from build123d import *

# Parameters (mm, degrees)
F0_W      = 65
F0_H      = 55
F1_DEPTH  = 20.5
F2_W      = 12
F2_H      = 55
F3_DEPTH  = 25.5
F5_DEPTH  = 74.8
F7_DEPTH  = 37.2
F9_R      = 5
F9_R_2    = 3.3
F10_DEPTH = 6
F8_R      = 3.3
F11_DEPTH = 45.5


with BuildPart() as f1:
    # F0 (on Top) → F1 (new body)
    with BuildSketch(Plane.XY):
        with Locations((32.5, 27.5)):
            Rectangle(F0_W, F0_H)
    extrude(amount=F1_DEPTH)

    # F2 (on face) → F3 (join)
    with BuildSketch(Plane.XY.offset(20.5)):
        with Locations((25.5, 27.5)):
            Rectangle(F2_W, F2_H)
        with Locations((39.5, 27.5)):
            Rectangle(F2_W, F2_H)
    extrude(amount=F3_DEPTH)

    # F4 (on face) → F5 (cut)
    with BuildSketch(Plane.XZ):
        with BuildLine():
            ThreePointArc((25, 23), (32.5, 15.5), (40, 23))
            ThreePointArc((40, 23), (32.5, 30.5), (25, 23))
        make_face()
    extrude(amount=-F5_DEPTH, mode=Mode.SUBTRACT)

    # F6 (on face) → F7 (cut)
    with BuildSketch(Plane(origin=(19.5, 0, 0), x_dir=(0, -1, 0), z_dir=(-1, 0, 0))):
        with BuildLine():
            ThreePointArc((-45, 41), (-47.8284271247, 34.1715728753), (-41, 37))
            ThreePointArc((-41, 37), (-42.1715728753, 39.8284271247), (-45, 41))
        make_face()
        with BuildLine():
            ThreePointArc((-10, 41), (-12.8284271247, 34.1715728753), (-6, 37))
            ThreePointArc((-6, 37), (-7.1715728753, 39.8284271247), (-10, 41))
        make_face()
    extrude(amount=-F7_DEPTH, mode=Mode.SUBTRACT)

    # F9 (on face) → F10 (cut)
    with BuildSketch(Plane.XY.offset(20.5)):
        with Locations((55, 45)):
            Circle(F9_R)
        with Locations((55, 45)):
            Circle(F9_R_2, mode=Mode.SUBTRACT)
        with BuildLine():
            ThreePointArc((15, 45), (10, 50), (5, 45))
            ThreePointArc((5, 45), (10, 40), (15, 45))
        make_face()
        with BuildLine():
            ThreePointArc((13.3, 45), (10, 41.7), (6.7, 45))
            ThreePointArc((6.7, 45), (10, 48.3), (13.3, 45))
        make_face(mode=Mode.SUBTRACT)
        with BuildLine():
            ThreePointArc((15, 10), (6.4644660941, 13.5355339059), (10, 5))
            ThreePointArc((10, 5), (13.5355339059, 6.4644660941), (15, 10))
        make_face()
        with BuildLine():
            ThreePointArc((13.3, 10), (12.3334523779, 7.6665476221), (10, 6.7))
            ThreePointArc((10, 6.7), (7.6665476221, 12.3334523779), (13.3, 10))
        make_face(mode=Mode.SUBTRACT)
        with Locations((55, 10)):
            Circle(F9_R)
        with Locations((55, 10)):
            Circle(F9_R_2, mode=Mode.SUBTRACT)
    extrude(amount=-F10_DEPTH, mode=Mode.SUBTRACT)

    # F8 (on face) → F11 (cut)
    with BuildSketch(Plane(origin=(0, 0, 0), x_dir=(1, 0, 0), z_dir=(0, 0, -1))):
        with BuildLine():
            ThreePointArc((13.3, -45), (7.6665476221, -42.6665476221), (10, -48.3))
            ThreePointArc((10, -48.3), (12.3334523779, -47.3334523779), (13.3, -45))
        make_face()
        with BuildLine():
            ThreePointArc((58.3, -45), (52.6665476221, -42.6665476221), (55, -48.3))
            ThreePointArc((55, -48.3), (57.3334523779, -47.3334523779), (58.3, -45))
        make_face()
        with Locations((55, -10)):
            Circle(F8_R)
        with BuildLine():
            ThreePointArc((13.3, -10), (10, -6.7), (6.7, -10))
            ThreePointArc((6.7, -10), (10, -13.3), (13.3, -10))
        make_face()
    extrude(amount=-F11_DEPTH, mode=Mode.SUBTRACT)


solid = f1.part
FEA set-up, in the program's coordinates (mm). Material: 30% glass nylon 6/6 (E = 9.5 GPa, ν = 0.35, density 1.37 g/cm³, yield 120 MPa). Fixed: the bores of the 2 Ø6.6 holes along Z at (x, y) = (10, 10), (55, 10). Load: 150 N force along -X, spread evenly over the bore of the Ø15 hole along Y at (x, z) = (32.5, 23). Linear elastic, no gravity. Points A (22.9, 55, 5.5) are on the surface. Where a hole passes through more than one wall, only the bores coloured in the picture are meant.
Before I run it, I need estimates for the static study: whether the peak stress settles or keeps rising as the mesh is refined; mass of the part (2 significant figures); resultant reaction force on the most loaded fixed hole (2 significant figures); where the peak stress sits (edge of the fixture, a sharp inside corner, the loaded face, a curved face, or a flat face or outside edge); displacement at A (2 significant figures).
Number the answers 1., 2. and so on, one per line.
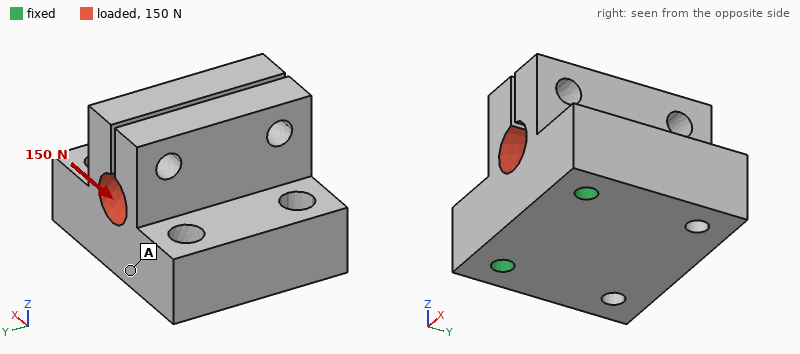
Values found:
1. keeps rising
2. 130 g
3. 100 N
4. edge of the fixture
5. 1.2 µm
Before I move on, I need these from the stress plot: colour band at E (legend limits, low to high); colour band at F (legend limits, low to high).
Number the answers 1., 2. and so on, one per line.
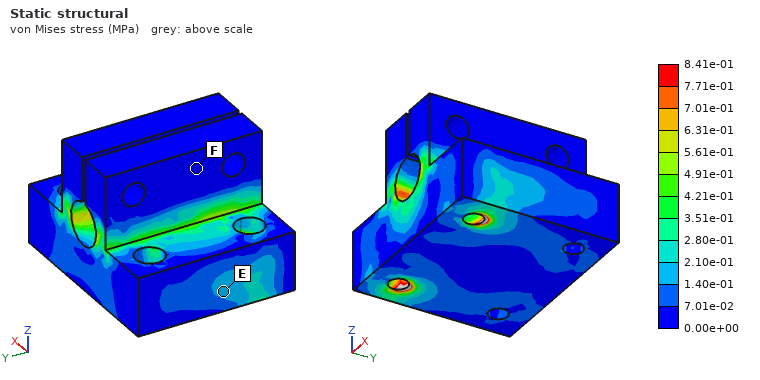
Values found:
1. 1.40e-01 to 2.10e-01 MPa
2. 0.00e+00 to 7.01e-02 MPa
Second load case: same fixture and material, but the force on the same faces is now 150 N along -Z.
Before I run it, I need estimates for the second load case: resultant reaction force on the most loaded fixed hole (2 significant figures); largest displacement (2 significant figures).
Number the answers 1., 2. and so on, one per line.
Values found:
1. 76 N
2. 14 µm
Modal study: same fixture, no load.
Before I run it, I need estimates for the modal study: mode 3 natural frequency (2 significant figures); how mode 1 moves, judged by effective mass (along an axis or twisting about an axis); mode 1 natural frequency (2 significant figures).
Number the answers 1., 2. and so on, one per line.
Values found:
1. 2300 Hz
2. along Z
3. 2000 Hz
